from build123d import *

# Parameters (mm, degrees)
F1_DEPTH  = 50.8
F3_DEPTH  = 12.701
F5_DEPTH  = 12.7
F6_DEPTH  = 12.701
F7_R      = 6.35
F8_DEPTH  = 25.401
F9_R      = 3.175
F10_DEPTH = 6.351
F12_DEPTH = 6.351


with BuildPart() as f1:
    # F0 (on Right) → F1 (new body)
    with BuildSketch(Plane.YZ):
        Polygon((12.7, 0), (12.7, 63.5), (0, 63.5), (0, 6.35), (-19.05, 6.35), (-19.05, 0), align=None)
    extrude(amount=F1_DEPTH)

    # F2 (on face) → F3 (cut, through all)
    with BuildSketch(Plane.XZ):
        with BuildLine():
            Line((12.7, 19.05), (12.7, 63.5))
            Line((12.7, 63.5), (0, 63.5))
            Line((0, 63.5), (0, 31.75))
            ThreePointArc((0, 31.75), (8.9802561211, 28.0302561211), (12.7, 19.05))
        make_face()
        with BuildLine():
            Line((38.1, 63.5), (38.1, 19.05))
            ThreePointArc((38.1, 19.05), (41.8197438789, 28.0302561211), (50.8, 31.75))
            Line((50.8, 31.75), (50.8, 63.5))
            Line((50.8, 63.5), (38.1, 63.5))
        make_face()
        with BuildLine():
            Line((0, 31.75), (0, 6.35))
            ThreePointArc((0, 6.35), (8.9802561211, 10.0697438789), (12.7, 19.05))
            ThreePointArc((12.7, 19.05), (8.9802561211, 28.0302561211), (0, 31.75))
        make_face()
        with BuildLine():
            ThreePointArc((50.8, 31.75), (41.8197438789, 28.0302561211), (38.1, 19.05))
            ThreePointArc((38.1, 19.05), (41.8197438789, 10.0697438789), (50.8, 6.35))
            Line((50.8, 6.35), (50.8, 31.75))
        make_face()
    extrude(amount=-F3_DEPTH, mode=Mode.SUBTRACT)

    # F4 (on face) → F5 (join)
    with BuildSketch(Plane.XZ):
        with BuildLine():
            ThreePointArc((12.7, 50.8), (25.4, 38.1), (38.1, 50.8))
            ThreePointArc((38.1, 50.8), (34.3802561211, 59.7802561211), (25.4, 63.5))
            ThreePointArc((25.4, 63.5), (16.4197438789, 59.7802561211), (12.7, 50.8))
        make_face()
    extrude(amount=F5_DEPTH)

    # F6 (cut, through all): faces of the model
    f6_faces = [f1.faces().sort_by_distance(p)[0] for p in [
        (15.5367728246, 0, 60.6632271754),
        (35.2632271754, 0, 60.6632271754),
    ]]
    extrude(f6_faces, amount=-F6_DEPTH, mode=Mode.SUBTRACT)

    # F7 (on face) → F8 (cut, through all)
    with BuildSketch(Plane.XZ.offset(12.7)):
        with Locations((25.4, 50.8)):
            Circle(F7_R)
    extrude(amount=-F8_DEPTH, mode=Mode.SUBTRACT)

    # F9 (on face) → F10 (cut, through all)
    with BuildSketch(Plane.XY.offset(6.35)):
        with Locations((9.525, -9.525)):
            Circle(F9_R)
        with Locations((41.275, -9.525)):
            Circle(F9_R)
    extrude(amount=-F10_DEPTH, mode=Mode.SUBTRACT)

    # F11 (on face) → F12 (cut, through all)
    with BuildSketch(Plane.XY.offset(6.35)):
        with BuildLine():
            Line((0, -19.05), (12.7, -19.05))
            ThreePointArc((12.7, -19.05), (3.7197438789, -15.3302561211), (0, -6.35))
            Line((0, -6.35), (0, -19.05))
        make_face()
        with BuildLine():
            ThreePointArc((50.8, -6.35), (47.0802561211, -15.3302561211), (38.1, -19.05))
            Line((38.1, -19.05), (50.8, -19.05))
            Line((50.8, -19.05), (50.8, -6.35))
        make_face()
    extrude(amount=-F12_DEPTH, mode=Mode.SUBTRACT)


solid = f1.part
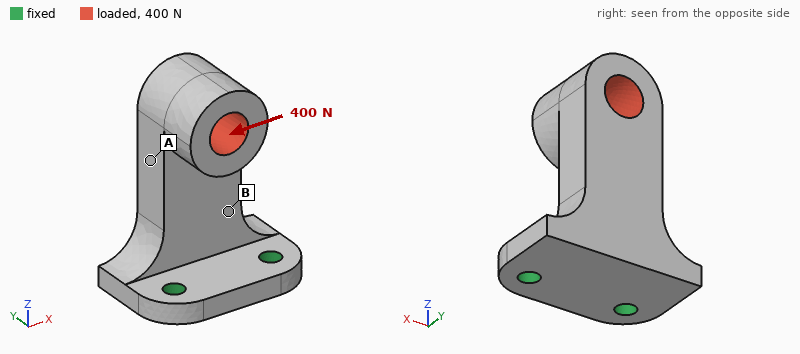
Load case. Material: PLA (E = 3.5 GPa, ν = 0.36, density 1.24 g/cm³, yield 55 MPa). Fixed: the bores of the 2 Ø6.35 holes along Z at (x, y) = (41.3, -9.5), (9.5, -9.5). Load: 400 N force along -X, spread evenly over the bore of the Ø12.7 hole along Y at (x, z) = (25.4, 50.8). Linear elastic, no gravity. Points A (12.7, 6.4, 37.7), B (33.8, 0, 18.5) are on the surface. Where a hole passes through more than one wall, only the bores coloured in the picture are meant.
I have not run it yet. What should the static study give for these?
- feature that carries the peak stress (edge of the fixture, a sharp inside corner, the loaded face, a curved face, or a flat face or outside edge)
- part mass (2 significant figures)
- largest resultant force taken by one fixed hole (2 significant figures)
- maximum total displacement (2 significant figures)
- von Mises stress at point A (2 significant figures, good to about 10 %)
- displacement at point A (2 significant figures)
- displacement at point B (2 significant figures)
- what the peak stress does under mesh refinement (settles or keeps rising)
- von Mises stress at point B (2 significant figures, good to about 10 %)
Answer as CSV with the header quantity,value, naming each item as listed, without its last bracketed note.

quantity,value
feature that carries the peak stress,edge of the fixture
part mass,39 g
largest resultant force taken by one fixed hole,610 N
maximum total displacement,1.0 mm
von Mises stress at point A,5.0 MPa
displacement at point A,0.48 mm
displacement at point B,0.21 mm
what the peak stress does under mesh refinement,keeps rising
von Mises stress at point B,11 MPa
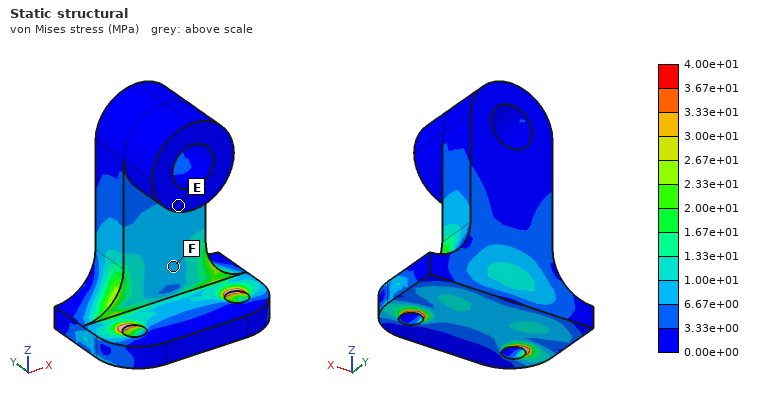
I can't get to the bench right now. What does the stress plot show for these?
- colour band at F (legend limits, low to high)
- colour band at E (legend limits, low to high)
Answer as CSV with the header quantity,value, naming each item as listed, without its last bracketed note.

quantity,value
colour band at F,6.67e+00 to 1.00e+01 MPa
colour band at E,0.00e+00 to 3.33e+00 MPa
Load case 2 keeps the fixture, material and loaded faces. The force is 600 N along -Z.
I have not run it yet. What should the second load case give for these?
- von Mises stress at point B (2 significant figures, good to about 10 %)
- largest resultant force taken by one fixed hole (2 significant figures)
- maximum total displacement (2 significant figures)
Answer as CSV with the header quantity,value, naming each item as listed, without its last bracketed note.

quantity,value
von Mises stress at point B,7.2 MPa
largest resultant force taken by one fixed hole,300 N
maximum total displacement,0.22 mm
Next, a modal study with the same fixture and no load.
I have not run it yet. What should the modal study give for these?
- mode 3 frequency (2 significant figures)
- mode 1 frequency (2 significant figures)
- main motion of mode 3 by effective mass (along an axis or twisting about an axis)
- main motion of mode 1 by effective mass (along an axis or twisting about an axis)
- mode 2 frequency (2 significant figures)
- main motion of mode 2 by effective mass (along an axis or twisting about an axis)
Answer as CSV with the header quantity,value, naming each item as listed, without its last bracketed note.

quantity,value
mode 3 frequency,2000 Hz
mode 1 frequency,410 Hz
main motion of mode 3 by effective mass,along Z
main motion of mode 1 by effective mass,along Y
mode 2 frequency,970 Hz
main motion of mode 2 by effective mass,along X
